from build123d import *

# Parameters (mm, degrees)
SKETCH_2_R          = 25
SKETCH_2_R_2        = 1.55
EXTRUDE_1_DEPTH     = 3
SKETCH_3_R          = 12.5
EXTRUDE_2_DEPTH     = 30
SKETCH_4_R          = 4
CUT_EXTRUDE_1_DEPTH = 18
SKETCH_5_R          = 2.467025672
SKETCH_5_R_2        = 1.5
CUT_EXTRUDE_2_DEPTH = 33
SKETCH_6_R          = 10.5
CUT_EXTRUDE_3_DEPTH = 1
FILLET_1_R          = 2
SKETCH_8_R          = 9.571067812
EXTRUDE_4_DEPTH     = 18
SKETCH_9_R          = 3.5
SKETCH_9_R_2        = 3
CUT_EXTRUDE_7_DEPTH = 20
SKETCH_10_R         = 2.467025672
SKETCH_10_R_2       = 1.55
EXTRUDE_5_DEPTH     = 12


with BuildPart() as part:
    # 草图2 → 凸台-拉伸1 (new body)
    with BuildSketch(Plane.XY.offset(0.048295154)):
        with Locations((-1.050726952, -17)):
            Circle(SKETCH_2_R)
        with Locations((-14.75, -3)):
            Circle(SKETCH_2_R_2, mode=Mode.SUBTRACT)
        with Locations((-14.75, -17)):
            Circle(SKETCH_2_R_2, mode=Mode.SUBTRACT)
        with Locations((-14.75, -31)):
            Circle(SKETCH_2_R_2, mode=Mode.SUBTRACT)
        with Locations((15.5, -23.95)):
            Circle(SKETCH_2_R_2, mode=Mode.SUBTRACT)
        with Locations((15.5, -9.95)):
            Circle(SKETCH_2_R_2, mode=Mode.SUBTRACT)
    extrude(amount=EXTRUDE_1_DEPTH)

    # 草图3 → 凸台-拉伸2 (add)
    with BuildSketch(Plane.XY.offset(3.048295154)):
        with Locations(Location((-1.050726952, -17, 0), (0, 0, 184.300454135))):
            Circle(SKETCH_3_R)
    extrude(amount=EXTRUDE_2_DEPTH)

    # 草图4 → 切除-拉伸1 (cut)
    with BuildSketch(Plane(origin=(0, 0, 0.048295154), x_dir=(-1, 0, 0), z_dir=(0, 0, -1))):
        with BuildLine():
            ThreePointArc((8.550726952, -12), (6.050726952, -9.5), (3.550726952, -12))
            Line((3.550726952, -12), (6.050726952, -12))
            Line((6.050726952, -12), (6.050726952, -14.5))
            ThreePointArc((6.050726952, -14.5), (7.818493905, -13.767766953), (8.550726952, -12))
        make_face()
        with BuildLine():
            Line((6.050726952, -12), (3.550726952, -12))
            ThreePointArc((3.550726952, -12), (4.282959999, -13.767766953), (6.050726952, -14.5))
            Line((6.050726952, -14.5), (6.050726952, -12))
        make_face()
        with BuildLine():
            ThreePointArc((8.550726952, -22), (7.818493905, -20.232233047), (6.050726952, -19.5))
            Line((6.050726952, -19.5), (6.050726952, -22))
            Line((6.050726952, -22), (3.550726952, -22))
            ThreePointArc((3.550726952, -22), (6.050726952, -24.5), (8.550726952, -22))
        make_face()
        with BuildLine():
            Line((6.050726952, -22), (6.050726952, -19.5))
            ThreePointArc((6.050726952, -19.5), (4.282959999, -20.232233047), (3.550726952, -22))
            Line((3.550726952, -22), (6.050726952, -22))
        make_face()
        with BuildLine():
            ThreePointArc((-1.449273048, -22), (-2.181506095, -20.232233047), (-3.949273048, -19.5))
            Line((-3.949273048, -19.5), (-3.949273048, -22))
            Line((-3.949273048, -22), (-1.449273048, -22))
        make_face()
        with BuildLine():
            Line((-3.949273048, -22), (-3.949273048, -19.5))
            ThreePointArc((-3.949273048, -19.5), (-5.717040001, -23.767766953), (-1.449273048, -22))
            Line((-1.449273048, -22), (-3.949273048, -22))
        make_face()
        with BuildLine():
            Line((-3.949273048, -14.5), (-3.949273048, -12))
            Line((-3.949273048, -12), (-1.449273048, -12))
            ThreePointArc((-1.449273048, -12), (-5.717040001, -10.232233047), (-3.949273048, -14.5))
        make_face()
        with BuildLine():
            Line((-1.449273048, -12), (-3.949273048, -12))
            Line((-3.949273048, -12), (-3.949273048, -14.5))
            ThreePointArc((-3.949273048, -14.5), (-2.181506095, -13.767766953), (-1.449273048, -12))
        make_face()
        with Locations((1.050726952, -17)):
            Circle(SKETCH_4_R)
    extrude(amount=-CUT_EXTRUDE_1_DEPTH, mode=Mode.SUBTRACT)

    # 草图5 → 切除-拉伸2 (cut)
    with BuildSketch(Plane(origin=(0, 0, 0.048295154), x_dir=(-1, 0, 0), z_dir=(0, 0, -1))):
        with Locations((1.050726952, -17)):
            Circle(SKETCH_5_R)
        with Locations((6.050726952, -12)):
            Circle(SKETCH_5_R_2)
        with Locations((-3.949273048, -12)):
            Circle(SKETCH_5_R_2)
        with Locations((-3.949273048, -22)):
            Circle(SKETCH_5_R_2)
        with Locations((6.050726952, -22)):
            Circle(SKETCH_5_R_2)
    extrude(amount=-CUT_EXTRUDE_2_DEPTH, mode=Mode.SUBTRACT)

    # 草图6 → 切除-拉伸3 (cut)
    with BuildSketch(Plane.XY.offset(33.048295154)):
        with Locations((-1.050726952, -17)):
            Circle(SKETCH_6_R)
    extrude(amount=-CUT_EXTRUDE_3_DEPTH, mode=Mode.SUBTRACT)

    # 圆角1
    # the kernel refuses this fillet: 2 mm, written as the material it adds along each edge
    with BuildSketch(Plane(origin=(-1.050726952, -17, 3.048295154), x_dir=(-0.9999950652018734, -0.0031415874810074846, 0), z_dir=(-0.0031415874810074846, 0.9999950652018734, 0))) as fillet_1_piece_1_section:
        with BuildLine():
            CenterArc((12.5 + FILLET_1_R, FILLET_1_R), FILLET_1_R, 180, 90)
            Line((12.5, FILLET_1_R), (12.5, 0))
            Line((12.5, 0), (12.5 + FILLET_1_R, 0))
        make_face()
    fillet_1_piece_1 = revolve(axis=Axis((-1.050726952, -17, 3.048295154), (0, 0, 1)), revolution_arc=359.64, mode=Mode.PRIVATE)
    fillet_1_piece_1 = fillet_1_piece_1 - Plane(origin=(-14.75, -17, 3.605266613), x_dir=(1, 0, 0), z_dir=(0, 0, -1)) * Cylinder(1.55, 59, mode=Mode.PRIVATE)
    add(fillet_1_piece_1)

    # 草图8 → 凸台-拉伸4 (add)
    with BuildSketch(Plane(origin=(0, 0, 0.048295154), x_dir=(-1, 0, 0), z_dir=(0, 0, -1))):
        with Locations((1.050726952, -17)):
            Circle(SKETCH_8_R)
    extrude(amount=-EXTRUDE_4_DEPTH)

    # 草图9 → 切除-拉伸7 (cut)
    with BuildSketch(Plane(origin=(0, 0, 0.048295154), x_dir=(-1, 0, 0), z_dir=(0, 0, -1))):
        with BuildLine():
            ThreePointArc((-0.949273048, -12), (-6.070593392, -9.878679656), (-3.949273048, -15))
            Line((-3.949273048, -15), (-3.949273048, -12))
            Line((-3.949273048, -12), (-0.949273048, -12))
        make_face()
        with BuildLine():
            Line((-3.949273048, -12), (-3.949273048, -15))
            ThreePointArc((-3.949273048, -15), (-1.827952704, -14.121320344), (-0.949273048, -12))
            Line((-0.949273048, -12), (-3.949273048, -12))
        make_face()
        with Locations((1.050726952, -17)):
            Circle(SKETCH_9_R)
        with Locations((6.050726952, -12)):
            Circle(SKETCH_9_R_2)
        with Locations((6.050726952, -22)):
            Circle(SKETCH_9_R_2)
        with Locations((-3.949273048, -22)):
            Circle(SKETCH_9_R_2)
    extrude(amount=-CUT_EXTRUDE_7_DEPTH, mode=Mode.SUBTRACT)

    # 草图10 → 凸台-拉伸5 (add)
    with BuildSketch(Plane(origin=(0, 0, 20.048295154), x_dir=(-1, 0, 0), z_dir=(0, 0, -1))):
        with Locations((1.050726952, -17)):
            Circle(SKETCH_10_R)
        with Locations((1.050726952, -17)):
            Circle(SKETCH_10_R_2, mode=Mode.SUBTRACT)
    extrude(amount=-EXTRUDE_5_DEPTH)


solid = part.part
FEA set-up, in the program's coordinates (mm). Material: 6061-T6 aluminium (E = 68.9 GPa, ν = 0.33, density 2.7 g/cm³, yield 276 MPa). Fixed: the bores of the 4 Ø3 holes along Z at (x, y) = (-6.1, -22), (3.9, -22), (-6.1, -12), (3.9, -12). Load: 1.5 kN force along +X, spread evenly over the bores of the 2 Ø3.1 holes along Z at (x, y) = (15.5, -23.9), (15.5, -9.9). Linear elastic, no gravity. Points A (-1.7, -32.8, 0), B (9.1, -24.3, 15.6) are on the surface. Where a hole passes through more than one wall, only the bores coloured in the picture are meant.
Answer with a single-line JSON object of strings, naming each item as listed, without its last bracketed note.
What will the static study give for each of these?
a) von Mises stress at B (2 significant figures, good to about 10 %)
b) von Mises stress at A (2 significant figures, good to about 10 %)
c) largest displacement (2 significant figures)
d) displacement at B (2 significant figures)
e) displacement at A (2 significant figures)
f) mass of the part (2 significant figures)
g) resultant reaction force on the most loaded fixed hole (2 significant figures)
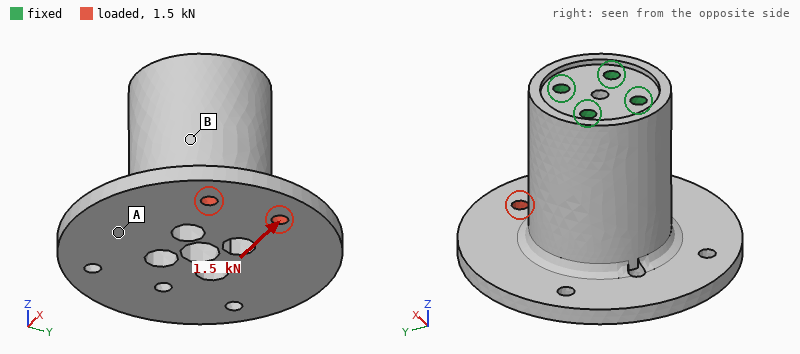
{"von Mises stress at B": "15 MPa", "von Mises stress at A": "5.8 MPa", "largest displacement": "29 µm", "displacement at B": "5.6 µm", "displacement at A": "15 µm", "mass of the part": "45 g", "resultant reaction force on the most loaded fixed hole": "1.0 kN"}
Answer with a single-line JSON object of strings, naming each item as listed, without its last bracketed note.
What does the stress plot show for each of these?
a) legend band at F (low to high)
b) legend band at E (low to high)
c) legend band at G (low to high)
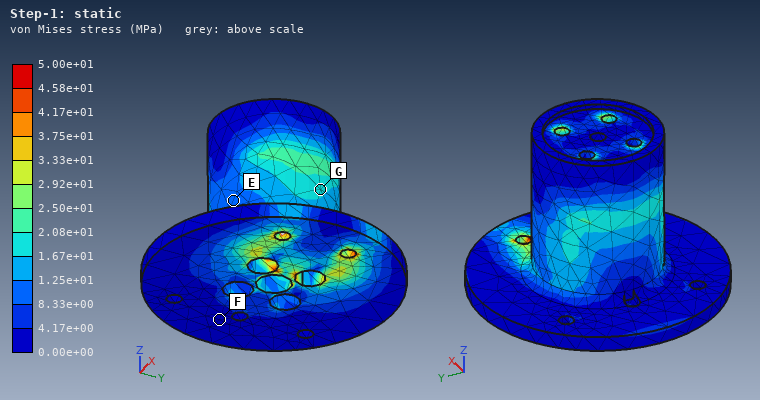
{"legend band at F": "0.00e+00 to 4.17e+00 MPa", "legend band at E": "8.33e+00 to 1.25e+01 MPa", "legend band at G": "1.67e+01 to 2.08e+01 MPa"}
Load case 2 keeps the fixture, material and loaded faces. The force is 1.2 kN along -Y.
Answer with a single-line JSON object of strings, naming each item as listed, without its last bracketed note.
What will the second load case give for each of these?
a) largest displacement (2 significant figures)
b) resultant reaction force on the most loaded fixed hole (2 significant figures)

{"largest displacement": "31 µm", "resultant reaction force on the most loaded fixed hole": "1.2 kN"}
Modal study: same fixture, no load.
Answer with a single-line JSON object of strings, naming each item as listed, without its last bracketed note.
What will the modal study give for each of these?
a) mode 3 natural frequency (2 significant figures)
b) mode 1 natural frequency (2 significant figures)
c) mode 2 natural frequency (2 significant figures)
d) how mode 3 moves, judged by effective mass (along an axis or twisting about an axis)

{"mode 3 natural frequency": "12 kHz", "mode 1 natural frequency": "9500 Hz", "mode 2 natural frequency": "9600 Hz", "how mode 3 moves, judged by effective mass": "along Z"}
